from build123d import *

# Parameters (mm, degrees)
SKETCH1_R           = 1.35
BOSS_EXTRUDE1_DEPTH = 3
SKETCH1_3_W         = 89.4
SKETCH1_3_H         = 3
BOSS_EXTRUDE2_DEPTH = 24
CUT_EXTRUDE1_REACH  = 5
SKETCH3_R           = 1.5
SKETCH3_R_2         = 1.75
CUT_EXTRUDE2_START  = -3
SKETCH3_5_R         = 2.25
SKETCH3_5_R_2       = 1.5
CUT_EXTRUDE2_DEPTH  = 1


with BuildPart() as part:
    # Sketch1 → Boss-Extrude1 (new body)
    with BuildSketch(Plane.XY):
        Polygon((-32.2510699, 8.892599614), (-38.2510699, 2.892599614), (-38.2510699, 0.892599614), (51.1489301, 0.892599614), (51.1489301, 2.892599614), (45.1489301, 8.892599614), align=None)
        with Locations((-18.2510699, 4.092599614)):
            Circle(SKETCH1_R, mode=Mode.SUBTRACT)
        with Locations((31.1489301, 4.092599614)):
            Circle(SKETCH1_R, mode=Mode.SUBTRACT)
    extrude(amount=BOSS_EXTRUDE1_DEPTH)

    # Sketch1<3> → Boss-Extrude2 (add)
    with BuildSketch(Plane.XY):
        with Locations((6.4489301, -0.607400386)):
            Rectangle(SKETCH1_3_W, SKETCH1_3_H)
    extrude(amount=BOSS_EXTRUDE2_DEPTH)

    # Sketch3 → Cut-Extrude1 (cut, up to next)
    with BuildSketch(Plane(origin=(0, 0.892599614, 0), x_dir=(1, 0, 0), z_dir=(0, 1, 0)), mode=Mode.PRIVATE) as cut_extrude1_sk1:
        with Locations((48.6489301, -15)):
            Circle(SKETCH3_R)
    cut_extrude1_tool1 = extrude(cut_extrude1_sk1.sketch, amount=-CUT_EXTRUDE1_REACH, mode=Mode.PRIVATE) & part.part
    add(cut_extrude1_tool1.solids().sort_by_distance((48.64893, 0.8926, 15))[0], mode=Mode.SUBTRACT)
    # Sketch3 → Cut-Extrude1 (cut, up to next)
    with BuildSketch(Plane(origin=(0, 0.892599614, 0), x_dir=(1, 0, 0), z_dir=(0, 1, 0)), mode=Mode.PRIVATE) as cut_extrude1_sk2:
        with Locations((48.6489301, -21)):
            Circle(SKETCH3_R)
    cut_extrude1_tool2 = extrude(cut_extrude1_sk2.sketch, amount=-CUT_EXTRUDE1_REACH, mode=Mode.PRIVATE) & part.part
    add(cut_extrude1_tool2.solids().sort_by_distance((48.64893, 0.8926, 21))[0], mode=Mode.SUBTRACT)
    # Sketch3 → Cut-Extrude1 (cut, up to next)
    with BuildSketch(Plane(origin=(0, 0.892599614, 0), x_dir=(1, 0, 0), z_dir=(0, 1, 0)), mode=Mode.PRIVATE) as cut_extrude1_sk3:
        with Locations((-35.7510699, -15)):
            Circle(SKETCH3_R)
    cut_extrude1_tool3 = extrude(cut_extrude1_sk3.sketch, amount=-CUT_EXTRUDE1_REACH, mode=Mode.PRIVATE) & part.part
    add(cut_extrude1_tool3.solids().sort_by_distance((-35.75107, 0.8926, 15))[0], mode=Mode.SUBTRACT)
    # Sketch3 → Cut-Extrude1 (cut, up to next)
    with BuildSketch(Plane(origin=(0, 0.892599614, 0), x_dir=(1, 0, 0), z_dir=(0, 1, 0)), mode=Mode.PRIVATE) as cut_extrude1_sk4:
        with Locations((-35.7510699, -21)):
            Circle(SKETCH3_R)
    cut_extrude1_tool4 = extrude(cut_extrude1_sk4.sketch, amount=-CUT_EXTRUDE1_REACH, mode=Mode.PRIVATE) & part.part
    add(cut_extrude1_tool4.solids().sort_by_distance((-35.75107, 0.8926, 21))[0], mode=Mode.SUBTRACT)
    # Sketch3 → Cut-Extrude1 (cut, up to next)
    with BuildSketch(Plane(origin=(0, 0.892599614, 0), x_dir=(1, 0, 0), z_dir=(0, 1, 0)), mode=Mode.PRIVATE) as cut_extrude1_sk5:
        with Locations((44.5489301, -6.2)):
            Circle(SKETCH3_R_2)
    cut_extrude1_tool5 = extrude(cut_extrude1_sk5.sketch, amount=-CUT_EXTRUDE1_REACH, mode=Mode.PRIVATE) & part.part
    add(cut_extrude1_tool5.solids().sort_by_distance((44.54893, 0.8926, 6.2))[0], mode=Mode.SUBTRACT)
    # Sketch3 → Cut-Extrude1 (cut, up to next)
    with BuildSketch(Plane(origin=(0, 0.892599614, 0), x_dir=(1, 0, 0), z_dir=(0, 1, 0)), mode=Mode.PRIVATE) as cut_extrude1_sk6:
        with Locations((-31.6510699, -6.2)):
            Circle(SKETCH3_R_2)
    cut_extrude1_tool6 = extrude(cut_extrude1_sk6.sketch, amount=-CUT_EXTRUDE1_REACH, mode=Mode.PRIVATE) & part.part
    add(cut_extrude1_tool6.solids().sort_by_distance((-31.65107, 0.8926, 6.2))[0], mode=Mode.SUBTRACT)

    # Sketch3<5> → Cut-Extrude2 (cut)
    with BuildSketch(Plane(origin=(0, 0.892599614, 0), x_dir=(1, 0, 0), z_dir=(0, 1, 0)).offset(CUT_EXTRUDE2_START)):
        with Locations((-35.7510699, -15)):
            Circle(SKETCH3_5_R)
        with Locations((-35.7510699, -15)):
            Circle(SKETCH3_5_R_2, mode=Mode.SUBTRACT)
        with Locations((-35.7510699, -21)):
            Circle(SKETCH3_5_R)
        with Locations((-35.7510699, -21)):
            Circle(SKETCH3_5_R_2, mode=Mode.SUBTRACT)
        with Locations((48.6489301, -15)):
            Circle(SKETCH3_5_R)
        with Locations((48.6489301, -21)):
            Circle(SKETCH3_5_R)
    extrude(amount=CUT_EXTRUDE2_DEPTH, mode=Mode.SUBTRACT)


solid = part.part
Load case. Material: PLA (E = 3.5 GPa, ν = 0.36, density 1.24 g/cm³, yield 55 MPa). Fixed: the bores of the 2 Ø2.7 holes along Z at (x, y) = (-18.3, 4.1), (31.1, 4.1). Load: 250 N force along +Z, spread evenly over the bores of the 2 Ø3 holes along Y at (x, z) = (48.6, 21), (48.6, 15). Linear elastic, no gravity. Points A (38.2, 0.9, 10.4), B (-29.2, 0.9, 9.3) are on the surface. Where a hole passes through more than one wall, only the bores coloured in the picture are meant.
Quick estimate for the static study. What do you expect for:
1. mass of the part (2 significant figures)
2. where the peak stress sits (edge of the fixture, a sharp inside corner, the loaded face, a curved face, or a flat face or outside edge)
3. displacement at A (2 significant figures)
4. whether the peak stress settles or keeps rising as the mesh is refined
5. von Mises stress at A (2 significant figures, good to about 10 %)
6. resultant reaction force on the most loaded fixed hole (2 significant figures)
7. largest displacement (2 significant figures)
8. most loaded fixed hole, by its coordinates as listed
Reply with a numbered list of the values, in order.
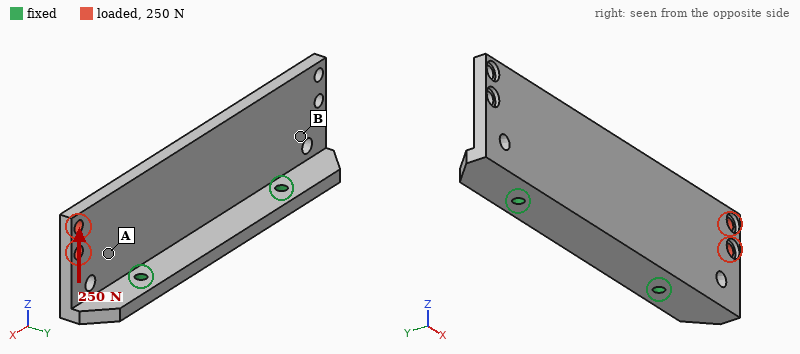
1. 10 g
2. edge of the fixture
3. 0.29 mm
4. keeps rising
5. 10 MPa
6. 340 N
7. 0.65 mm
8. (31.1, 4.1)
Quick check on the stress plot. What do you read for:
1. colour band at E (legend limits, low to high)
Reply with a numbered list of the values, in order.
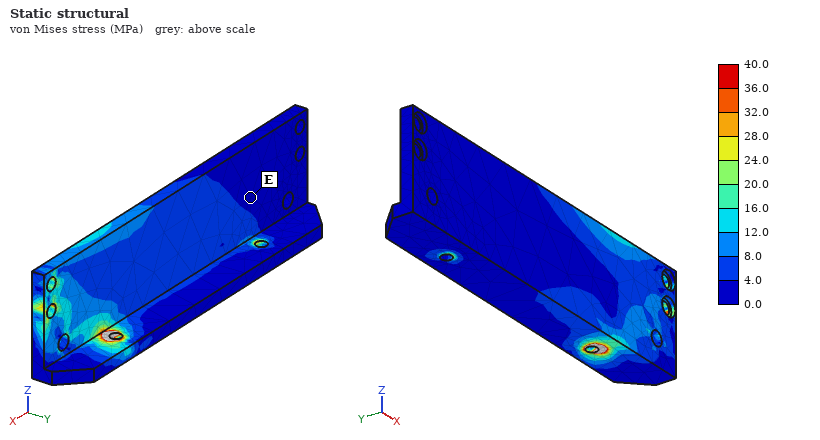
1. 0.0 to 4.0 MPa
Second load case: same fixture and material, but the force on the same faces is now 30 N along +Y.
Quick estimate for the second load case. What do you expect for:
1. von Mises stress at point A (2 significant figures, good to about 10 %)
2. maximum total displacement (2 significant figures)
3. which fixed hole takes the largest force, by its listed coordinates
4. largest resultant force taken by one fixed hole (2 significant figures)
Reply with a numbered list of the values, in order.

1. 7.7 MPa
2. 0.98 mm
3. (31.1, 4.1)
4. 39 N
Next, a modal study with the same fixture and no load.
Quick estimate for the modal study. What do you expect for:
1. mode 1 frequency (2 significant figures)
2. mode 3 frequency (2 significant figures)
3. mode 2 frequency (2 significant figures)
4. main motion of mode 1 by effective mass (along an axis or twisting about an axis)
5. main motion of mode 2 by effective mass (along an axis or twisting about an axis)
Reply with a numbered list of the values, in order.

1. 920 Hz
2. 1800 Hz
3. 1300 Hz
4. along Y
5. twisting about Z
